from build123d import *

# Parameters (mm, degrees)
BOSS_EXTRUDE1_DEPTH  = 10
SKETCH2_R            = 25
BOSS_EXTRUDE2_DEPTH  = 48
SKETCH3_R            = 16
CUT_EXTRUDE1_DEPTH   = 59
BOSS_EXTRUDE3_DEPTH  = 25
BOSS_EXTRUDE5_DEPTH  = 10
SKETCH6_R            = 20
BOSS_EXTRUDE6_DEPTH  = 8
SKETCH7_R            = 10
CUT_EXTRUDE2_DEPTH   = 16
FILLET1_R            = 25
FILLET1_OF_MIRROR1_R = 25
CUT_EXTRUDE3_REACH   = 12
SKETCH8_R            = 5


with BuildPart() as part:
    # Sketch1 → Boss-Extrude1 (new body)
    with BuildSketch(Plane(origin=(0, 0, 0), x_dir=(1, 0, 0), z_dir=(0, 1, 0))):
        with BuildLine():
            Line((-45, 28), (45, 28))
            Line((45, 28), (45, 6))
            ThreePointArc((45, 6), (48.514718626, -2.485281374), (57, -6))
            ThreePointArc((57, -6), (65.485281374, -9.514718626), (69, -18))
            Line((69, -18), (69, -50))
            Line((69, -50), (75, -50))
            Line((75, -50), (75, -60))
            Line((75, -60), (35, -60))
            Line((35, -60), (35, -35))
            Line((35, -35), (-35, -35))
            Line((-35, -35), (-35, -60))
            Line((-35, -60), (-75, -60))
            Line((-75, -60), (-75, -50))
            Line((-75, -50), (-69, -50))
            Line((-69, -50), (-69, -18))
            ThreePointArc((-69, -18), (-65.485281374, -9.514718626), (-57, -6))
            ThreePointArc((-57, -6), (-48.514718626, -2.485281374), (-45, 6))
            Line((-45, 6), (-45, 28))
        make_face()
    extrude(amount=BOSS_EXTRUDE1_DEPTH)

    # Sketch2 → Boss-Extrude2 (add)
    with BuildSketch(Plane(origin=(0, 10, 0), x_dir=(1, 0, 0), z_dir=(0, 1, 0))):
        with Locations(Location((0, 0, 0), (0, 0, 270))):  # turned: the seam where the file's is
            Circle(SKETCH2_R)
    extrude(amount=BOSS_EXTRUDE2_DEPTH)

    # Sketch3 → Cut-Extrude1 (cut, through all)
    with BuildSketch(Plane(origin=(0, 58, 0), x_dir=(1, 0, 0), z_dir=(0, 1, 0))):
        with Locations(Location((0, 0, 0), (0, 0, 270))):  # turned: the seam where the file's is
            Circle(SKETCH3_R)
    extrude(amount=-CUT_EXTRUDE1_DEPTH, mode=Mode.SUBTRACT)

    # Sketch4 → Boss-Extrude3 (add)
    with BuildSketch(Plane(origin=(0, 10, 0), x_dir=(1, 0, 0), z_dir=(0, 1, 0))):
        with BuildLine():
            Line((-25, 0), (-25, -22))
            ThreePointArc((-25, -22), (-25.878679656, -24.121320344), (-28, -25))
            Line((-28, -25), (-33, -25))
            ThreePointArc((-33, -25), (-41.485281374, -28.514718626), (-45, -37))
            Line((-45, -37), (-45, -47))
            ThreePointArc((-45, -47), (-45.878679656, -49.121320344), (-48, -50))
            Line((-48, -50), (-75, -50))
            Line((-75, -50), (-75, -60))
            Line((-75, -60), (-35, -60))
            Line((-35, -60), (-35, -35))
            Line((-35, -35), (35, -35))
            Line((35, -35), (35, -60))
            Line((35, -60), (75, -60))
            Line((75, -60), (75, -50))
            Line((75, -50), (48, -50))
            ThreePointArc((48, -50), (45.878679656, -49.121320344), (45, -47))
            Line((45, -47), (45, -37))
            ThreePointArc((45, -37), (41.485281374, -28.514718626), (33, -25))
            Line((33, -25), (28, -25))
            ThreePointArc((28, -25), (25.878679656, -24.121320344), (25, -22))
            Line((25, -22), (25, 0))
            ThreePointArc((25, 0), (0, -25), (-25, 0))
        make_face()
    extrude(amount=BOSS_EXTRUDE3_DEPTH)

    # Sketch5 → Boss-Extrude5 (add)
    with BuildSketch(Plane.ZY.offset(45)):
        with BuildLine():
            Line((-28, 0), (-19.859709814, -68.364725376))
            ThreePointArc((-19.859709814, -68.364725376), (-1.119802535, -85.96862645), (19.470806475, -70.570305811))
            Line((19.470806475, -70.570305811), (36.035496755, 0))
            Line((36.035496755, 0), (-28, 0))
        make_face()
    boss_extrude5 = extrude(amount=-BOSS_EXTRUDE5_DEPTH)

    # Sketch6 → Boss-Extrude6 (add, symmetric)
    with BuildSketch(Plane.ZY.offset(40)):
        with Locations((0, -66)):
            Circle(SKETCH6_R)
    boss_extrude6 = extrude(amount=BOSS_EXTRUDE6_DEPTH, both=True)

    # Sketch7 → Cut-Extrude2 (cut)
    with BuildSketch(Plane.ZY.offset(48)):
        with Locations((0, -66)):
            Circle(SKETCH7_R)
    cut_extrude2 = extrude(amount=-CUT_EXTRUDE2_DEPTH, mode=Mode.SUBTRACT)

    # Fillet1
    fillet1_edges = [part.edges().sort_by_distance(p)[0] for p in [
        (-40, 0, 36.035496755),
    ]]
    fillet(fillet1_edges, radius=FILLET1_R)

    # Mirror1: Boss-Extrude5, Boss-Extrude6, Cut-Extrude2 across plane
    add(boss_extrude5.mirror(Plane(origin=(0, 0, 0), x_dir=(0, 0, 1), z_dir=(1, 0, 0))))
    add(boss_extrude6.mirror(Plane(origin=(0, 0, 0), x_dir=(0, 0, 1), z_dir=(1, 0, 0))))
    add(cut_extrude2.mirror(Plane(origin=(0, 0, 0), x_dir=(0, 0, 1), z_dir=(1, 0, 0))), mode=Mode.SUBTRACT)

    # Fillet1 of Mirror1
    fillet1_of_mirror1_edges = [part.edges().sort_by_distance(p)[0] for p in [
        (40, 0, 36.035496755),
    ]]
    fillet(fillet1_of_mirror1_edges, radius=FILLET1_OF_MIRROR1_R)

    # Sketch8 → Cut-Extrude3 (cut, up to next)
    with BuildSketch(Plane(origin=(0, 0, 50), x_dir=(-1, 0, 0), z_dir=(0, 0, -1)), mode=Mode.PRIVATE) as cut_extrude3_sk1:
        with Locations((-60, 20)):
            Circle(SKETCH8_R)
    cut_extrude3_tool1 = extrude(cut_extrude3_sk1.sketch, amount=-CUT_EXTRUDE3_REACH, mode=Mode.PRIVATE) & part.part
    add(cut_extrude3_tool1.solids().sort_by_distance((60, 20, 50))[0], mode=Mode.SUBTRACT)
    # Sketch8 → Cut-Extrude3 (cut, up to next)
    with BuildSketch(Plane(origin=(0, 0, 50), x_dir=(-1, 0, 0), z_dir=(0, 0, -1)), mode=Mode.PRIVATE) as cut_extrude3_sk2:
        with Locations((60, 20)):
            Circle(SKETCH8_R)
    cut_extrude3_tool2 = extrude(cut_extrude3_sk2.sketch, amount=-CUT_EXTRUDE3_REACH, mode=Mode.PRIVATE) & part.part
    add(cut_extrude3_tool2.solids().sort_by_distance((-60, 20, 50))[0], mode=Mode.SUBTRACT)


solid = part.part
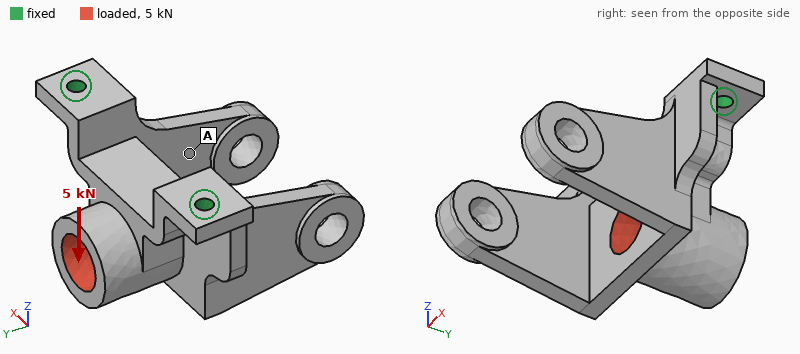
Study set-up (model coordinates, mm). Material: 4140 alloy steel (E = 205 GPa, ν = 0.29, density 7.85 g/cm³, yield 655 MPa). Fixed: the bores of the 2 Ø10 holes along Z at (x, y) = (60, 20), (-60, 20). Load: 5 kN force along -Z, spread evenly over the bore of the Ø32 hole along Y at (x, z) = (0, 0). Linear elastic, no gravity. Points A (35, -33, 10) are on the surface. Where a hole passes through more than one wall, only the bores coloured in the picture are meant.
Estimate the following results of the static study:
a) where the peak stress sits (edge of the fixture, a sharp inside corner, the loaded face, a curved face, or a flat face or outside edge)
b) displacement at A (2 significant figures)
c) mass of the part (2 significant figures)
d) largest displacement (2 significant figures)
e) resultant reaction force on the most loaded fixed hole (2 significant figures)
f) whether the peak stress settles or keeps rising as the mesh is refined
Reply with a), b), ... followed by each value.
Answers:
a) edge of the fixture
b) 30 µm
c) 2.2 kg
d) 59 µm
e) 3.0 kN
f) keeps rising
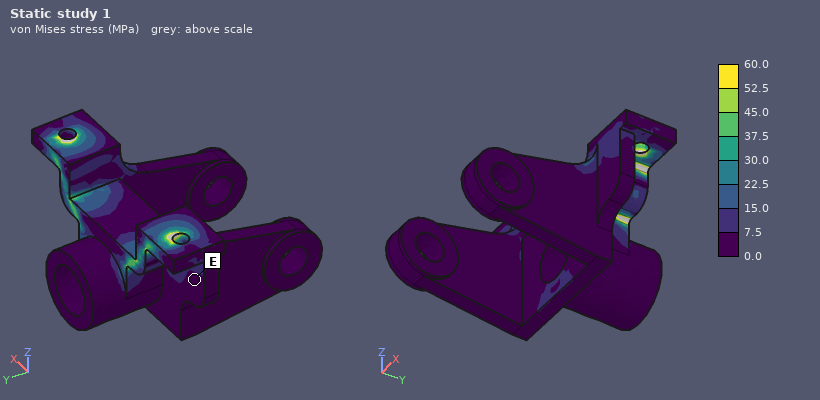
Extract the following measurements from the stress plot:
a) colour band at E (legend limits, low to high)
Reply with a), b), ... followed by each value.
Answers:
a) 0.0 to 7.5 MPa
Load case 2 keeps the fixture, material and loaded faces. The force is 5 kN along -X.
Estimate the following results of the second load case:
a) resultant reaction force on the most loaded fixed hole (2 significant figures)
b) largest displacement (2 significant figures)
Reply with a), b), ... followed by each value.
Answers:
a) 3.5 kN
b) 19 µm
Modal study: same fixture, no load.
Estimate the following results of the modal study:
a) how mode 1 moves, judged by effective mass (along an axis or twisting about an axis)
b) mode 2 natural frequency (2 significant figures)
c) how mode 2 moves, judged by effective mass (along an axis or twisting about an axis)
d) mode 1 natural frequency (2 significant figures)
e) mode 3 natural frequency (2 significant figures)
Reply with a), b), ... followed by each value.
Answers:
a) along Y
b) 960 Hz
c) along X
d) 680 Hz
e) 1000 Hz
